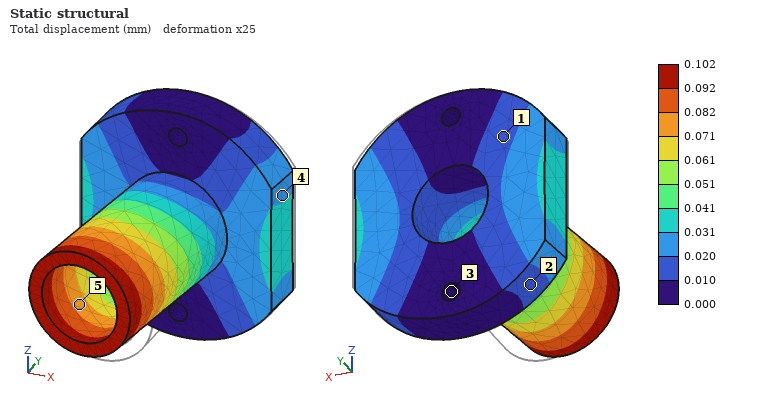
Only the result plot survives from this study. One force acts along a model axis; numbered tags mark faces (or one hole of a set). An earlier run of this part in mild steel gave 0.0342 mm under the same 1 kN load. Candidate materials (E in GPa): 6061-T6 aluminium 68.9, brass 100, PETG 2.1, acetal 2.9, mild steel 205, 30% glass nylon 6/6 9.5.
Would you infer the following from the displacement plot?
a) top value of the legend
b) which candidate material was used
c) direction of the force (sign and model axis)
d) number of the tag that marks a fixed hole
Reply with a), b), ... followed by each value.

a) 0.102 mm
b) 6061-T6 aluminium
c) -X
d) 3
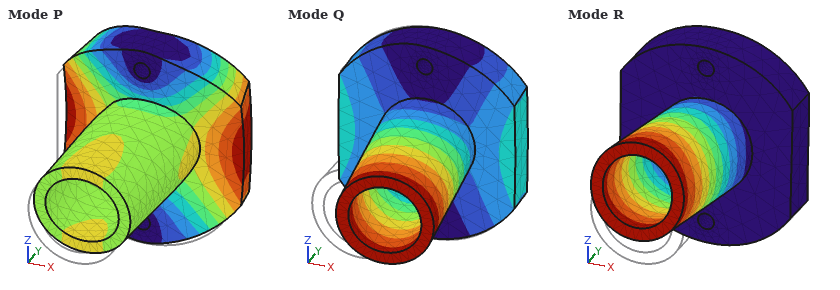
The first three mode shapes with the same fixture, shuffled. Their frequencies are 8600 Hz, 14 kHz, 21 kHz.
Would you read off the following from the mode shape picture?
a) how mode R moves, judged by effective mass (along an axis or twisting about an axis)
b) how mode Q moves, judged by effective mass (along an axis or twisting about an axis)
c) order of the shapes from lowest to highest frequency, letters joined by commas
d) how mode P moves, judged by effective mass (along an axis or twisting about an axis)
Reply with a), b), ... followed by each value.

a) along Z
b) along X
c) Q, R, P
d) along Y
